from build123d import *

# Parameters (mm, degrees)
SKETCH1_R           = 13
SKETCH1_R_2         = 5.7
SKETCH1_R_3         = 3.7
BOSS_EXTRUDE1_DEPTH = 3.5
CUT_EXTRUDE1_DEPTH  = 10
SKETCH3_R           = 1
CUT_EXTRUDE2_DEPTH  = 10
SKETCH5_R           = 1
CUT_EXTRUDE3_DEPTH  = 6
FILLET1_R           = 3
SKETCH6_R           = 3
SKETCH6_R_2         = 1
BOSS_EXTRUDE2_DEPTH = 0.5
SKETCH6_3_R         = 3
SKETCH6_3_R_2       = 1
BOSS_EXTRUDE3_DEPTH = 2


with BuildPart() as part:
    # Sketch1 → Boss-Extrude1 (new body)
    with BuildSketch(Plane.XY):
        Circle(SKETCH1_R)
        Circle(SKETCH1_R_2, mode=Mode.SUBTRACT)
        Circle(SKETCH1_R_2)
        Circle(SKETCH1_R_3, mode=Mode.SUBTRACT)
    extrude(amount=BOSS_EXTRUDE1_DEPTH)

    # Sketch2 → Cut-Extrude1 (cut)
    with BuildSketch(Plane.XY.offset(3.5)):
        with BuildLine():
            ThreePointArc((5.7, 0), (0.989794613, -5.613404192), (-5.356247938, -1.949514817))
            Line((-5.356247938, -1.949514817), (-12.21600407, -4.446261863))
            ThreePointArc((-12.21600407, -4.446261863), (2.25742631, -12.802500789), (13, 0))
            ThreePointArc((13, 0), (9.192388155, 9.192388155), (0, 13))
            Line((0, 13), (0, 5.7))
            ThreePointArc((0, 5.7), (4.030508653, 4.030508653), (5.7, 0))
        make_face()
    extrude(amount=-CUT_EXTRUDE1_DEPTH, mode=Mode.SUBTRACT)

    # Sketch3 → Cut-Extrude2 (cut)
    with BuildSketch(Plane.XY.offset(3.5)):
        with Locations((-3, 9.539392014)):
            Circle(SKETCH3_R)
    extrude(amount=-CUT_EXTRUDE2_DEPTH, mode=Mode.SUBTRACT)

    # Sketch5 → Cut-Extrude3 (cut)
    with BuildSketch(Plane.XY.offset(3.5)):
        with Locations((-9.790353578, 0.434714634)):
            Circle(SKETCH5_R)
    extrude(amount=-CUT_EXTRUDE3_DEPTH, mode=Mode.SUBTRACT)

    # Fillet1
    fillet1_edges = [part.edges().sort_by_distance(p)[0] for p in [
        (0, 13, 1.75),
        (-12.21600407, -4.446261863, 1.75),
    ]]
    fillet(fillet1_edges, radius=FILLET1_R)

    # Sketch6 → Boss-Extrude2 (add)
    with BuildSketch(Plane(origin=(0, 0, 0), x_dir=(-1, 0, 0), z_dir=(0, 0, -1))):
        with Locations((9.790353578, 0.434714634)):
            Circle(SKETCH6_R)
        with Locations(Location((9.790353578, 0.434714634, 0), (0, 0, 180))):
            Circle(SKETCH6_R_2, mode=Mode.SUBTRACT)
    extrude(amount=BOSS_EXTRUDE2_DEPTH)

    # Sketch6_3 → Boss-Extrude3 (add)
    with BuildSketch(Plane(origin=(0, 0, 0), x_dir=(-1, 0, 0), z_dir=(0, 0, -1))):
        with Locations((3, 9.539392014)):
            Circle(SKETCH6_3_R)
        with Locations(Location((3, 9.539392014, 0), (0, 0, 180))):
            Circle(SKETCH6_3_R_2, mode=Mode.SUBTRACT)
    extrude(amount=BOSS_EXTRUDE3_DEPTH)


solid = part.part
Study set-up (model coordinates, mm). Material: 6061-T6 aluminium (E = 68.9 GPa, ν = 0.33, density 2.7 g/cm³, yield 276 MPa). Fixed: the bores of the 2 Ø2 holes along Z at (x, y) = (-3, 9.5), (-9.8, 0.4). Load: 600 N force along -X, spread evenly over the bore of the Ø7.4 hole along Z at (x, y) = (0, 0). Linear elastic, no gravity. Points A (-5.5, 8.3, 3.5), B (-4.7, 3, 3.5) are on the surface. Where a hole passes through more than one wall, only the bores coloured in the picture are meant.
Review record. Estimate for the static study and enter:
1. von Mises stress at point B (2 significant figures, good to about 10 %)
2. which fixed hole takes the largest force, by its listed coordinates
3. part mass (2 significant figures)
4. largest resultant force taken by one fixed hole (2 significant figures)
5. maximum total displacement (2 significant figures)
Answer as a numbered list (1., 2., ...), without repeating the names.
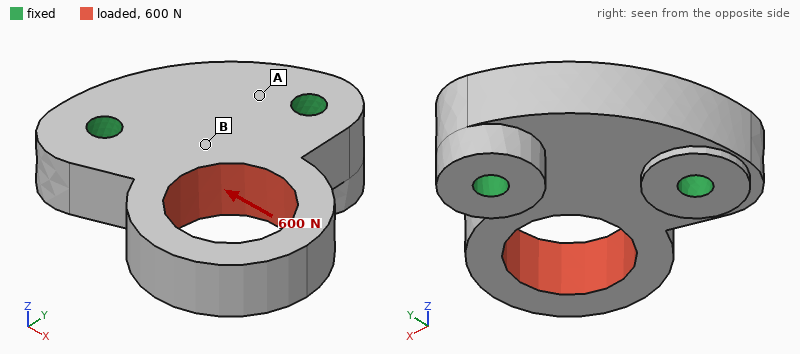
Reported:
1. 27 MPa
2. (-9.8, 0.4)
3. 1.9 g
4. 530 N
5. 30 µm
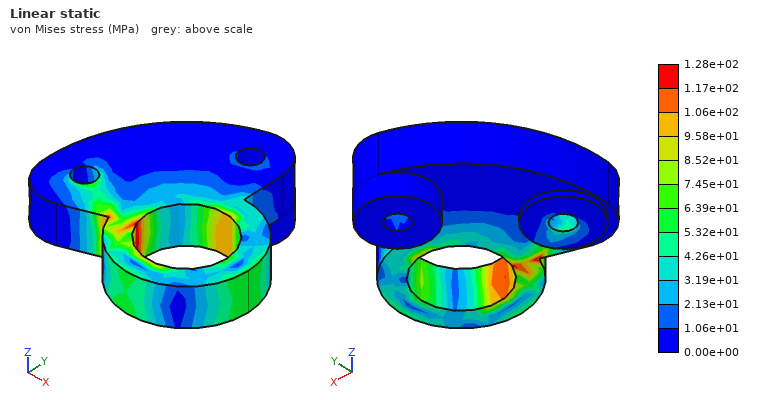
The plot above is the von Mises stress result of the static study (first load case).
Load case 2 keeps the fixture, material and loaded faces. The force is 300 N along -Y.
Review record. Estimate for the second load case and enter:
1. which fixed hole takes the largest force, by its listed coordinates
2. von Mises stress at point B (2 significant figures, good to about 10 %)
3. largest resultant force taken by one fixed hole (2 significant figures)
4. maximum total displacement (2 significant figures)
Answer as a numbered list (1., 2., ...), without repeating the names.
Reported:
1. (-3, 9.5)
2. 17 MPa
3. 280 N
4. 21 µm
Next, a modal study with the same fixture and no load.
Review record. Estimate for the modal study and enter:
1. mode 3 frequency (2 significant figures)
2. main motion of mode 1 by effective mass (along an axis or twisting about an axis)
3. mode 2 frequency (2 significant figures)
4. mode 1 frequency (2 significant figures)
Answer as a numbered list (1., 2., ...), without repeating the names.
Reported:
1. 38 kHz
2. along Z
3. 25 kHz
4. 17 kHz
